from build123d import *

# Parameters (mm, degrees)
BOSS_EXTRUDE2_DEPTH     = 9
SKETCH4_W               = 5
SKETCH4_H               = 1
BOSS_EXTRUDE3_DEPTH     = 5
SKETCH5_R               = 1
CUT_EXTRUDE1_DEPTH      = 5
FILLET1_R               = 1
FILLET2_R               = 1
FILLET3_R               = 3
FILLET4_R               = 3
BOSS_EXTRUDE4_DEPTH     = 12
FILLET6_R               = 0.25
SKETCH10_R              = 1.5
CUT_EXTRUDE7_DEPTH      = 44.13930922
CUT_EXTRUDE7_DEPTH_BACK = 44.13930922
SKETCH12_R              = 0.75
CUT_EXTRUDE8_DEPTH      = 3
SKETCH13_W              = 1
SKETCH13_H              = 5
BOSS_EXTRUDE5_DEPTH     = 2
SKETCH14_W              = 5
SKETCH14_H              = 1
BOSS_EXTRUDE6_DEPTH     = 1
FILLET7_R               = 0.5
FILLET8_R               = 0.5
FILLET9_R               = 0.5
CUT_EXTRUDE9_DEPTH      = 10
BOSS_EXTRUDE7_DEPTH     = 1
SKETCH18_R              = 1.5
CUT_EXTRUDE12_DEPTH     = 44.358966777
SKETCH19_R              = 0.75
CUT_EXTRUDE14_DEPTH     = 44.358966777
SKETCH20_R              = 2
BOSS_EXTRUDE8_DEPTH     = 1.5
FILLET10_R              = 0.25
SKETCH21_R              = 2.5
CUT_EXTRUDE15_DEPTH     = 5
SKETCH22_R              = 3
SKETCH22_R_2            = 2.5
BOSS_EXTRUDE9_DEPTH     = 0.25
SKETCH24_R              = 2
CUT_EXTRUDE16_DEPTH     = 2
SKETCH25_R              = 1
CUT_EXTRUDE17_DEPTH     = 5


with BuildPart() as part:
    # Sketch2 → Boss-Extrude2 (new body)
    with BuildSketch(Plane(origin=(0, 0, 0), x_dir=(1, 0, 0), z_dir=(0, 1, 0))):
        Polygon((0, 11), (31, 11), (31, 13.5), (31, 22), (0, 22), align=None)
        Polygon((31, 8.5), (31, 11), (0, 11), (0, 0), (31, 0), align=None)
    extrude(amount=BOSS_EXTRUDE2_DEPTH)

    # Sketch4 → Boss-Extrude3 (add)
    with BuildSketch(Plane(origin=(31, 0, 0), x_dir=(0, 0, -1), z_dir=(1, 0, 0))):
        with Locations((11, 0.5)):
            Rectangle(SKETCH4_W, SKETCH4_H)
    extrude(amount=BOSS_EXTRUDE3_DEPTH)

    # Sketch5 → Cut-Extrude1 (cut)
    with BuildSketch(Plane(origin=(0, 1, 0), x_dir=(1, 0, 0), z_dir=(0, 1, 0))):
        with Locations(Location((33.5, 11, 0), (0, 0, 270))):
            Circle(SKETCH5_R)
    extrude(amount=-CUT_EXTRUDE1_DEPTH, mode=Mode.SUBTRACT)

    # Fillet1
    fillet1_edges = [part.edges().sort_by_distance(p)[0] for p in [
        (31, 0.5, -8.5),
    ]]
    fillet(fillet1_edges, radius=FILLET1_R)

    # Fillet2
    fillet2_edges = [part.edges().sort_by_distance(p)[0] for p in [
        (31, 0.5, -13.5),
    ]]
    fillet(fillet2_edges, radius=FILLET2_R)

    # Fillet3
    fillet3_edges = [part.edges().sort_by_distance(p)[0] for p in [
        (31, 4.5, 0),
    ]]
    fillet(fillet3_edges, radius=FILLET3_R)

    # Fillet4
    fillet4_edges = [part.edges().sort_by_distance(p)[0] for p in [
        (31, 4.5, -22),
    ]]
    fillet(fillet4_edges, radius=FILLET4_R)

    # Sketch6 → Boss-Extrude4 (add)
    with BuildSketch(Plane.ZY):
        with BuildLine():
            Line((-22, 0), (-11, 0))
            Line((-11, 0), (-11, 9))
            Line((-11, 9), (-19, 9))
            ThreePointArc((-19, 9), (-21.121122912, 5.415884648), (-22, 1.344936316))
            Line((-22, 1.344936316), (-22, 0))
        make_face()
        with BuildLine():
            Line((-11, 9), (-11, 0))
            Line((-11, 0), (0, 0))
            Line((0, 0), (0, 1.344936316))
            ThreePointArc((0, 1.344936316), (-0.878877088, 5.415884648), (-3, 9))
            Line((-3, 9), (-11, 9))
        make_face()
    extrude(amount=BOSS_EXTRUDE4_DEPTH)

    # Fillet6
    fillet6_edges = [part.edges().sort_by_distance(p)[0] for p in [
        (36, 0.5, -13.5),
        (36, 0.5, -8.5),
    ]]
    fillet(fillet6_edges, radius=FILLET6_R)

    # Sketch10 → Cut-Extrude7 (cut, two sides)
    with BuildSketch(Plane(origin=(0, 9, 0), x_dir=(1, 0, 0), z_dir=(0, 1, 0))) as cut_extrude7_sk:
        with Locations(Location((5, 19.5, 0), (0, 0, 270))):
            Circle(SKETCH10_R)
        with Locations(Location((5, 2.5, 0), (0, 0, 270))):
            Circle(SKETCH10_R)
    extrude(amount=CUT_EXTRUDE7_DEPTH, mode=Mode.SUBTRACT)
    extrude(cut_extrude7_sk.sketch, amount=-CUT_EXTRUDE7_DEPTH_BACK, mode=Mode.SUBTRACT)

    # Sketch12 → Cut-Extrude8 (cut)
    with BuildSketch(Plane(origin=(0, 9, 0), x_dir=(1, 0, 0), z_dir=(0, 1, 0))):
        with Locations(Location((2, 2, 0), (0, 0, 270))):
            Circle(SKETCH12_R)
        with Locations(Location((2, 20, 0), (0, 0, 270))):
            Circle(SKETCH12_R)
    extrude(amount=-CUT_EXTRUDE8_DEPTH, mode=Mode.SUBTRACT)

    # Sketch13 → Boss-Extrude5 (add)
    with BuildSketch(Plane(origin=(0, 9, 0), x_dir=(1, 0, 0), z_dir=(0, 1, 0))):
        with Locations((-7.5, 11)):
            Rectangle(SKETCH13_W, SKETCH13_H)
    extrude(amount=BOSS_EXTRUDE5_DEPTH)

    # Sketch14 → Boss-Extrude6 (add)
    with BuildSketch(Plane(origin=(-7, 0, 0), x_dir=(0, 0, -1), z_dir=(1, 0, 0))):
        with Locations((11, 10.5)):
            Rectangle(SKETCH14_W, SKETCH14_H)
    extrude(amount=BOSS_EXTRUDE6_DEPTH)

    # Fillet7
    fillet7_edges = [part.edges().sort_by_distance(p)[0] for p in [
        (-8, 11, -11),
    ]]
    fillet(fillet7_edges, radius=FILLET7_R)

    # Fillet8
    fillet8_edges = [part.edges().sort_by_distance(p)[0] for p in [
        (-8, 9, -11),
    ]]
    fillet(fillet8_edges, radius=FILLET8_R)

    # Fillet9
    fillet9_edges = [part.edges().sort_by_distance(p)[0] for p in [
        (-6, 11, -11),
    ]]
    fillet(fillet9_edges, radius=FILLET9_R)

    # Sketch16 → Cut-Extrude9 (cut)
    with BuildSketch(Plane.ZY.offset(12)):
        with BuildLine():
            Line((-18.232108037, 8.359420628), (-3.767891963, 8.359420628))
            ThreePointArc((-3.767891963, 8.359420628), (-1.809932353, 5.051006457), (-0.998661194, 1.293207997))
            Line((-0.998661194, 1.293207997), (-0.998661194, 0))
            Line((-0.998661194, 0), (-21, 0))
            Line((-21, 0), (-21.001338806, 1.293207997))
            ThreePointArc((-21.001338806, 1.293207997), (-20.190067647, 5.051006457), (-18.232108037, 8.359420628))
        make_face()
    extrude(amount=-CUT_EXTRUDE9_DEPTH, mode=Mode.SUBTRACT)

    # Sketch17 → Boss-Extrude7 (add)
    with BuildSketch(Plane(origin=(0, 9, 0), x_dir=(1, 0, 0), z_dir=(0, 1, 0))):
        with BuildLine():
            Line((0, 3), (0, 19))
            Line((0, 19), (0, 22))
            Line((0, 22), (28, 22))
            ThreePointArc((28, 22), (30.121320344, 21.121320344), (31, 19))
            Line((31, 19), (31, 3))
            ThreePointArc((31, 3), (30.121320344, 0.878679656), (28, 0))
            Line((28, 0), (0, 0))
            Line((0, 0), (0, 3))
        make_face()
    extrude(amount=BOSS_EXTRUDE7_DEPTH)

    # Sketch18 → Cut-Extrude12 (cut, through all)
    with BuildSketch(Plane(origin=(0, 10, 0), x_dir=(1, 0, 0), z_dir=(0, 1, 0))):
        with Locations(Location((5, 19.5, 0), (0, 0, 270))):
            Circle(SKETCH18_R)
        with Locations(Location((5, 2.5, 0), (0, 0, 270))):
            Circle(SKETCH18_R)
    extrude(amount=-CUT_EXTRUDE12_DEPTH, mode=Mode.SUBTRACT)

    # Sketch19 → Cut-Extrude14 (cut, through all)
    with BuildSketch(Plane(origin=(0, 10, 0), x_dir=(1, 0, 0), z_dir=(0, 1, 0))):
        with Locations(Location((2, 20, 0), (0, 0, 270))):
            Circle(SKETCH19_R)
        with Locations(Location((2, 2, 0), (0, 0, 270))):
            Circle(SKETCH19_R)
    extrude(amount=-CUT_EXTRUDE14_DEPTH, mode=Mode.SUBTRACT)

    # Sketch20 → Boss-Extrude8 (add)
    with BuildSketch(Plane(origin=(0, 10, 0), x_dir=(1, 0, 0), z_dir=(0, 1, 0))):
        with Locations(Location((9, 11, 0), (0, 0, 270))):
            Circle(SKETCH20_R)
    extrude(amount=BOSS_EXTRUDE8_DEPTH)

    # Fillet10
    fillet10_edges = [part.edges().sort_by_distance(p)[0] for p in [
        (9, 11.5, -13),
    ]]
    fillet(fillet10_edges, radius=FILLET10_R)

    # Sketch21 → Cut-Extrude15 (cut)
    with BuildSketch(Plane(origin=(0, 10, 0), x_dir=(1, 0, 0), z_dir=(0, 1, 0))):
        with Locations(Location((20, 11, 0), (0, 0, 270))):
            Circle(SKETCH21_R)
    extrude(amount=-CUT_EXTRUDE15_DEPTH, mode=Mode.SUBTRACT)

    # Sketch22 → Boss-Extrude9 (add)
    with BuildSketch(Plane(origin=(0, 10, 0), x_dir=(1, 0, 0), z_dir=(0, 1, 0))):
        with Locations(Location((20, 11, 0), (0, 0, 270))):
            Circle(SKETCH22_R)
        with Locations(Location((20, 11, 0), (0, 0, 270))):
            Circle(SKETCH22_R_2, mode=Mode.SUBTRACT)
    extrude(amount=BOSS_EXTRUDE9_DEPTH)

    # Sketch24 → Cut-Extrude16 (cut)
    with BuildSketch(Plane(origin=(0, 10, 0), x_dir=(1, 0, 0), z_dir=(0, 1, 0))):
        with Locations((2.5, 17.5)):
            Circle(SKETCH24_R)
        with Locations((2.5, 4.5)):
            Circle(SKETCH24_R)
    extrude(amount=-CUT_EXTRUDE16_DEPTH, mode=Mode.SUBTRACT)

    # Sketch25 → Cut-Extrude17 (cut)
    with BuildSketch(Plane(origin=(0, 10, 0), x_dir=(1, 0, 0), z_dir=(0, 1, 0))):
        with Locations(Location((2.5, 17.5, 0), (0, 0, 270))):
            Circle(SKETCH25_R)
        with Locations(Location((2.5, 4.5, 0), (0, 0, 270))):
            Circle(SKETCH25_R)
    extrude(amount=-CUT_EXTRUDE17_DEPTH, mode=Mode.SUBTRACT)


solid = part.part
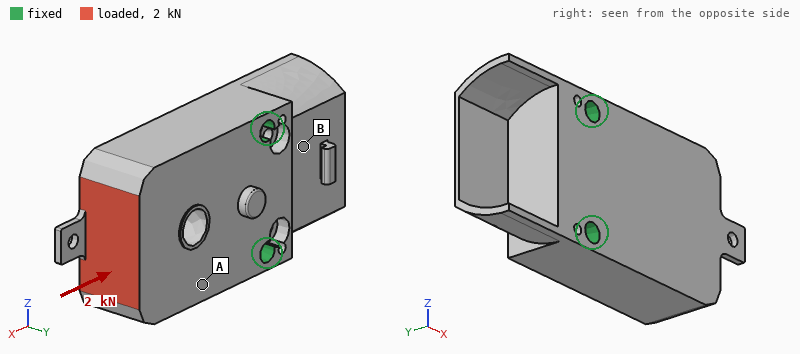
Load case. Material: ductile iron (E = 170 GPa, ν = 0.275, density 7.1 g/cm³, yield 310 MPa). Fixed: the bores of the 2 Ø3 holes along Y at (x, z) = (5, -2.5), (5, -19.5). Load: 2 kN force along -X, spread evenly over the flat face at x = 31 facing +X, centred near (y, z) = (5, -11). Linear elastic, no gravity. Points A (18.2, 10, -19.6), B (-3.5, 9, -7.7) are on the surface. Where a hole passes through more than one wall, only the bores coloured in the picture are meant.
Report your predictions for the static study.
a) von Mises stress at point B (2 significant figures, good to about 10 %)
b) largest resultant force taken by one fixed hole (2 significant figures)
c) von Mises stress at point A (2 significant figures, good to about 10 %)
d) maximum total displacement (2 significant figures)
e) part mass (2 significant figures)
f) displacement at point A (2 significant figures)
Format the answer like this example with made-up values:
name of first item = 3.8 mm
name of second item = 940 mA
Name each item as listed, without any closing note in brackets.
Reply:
von Mises stress at point B = 3.1 MPa
largest resultant force taken by one fixed hole = 1.0 kN
von Mises stress at point A = 11 MPa
maximum total displacement = 2.4 µm
part mass = 51 g
displacement at point A = 1.0 µm
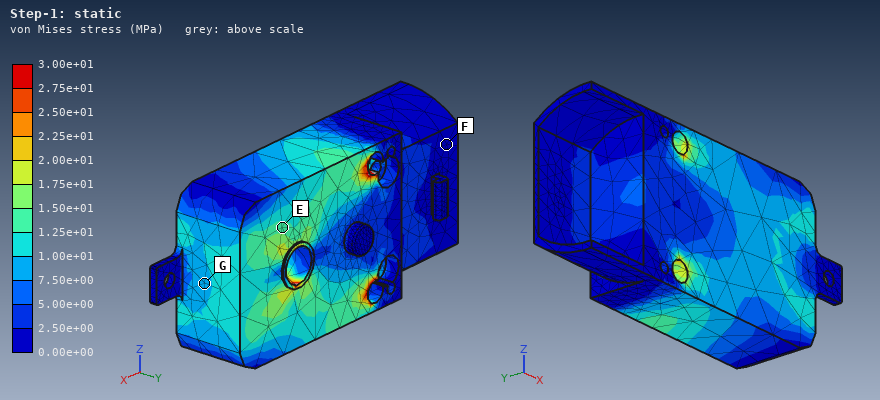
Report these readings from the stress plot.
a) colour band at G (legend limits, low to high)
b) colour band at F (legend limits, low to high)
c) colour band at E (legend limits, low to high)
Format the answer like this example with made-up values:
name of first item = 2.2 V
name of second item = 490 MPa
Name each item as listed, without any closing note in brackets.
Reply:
colour band at G = 7.50e+00 to 1.00e+01 MPa
colour band at F = 0.00e+00 to 2.50e+00 MPa
colour band at E = 1.25e+01 to 1.50e+01 MPa
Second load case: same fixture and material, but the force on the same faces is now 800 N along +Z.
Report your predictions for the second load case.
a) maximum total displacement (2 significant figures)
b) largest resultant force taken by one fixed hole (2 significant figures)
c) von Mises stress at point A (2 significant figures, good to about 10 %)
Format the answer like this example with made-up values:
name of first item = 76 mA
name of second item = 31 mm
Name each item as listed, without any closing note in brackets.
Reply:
maximum total displacement = 5.2 µm
largest resultant force taken by one fixed hole = 1.2 kN
von Mises stress at point A = 12 MPa
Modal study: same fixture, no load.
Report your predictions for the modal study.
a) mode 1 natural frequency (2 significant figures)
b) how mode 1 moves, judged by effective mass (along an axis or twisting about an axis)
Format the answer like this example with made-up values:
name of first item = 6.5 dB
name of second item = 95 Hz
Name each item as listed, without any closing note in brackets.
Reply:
mode 1 natural frequency = 9800 Hz
how mode 1 moves, judged by effective mass = along Y
